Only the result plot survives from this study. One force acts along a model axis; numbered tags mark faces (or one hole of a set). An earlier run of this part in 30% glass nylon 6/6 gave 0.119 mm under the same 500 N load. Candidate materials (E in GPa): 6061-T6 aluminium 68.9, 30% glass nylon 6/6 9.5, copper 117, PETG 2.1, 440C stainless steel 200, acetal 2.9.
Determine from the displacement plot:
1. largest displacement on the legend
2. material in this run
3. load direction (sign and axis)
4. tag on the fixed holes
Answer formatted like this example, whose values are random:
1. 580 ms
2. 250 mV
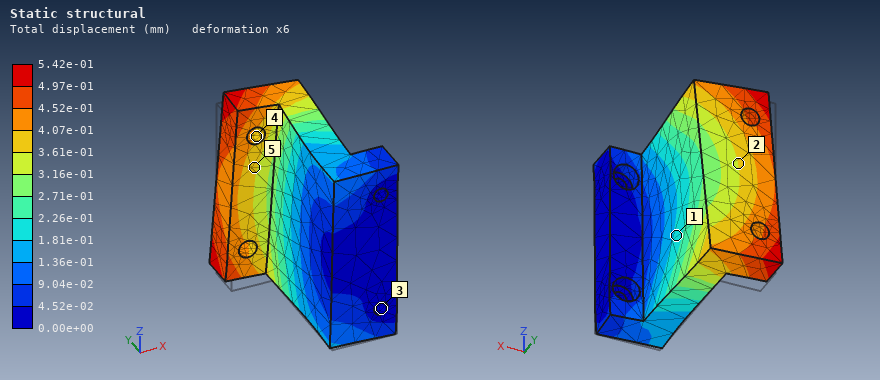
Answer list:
1. 5.42e-01 mm
2. PETG
3. +Z
4. 3
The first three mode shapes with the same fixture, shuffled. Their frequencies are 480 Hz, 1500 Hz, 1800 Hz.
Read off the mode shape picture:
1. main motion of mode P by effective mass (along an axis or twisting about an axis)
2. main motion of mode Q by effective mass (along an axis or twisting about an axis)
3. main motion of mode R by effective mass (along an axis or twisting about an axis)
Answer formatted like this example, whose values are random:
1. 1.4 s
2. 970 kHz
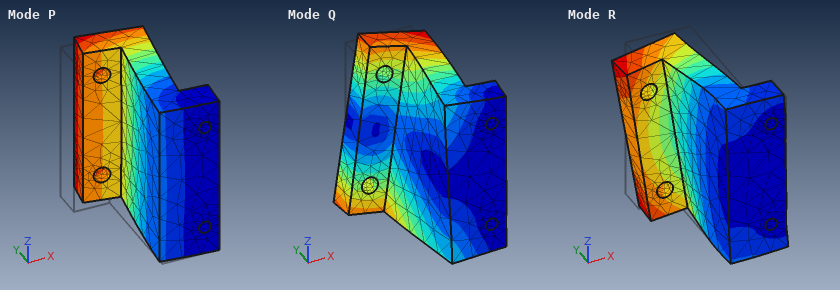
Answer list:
1. along X
2. along Z
3. along Z
